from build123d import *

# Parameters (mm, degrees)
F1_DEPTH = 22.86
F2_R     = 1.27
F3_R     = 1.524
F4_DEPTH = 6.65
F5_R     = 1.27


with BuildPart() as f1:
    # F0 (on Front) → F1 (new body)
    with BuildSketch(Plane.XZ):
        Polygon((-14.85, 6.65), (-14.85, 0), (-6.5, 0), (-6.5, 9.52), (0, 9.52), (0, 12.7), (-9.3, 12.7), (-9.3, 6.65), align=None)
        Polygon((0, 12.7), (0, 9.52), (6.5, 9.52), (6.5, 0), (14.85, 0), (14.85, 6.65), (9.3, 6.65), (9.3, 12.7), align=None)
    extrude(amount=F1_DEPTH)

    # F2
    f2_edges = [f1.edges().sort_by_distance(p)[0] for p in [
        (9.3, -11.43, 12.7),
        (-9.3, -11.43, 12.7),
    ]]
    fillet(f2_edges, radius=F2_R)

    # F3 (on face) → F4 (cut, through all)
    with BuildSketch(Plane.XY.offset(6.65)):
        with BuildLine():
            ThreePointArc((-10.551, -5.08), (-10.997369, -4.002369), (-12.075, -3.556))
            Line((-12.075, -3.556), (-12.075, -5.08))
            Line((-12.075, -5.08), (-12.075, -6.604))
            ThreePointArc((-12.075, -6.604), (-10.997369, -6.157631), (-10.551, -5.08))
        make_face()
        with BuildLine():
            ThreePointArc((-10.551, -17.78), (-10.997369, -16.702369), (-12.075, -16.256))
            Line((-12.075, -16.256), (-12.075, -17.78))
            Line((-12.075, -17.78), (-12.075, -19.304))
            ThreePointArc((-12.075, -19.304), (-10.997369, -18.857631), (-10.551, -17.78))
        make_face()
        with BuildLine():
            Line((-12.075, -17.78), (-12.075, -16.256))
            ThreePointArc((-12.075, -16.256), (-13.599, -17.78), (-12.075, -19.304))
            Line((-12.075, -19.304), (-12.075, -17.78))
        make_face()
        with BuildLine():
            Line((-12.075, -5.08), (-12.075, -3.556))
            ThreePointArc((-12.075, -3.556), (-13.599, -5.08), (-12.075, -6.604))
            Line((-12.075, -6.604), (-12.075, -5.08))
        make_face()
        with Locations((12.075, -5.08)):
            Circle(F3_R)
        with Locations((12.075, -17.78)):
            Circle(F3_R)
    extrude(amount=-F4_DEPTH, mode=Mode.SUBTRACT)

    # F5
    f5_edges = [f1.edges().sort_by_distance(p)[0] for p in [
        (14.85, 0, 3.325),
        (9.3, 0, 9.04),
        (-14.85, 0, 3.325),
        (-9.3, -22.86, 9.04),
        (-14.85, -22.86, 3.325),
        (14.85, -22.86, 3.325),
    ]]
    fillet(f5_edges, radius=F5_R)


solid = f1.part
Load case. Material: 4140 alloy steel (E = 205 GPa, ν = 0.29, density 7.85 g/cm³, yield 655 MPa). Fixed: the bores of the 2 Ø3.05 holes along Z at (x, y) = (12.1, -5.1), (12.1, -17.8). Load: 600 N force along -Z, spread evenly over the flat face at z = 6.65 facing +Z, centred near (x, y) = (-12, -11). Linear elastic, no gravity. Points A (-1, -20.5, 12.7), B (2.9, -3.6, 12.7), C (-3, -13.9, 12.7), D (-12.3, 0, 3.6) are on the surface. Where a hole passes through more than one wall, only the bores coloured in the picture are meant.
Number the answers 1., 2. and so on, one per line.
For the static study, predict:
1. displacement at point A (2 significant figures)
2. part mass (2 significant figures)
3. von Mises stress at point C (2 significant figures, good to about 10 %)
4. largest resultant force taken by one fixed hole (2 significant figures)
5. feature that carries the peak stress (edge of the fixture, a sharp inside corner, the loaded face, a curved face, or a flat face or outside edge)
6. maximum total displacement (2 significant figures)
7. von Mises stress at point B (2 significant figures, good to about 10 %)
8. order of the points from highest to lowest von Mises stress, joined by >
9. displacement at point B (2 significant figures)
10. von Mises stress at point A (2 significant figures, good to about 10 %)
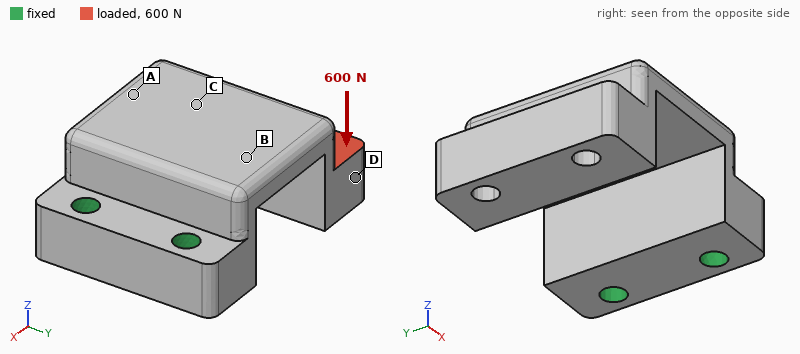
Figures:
1. 0.11 mm
2. 32 g
3. 130 MPa
4. 300 N
5. a sharp inside corner
6. 0.36 mm
7. 230 MPa
8. B > A > C > D
9. 0.067 mm
10. 180 MPa
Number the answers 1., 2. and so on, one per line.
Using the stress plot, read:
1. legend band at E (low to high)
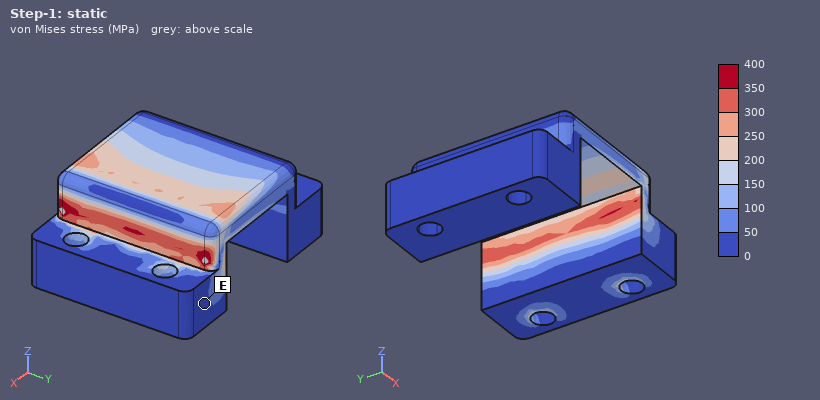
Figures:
1. 0 to 50 MPa
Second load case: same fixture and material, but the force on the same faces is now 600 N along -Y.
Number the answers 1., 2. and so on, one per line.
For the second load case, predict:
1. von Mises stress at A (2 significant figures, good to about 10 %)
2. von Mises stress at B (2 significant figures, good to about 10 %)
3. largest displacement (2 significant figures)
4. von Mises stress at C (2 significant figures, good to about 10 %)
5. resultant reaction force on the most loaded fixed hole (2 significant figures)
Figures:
1. 49 MPa
2. 65 MPa
3. 71 µm
4. 29 MPa
5. 1000 N
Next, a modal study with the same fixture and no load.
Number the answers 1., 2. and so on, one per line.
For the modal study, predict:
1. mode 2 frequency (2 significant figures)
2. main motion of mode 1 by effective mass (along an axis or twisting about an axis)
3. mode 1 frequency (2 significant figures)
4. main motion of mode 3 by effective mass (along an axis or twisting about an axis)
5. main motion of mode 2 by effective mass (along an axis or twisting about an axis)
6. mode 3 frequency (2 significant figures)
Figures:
1. 4300 Hz
2. along Z
3. 2200 Hz
4. along X
5. along Y
6. 7400 Hz
